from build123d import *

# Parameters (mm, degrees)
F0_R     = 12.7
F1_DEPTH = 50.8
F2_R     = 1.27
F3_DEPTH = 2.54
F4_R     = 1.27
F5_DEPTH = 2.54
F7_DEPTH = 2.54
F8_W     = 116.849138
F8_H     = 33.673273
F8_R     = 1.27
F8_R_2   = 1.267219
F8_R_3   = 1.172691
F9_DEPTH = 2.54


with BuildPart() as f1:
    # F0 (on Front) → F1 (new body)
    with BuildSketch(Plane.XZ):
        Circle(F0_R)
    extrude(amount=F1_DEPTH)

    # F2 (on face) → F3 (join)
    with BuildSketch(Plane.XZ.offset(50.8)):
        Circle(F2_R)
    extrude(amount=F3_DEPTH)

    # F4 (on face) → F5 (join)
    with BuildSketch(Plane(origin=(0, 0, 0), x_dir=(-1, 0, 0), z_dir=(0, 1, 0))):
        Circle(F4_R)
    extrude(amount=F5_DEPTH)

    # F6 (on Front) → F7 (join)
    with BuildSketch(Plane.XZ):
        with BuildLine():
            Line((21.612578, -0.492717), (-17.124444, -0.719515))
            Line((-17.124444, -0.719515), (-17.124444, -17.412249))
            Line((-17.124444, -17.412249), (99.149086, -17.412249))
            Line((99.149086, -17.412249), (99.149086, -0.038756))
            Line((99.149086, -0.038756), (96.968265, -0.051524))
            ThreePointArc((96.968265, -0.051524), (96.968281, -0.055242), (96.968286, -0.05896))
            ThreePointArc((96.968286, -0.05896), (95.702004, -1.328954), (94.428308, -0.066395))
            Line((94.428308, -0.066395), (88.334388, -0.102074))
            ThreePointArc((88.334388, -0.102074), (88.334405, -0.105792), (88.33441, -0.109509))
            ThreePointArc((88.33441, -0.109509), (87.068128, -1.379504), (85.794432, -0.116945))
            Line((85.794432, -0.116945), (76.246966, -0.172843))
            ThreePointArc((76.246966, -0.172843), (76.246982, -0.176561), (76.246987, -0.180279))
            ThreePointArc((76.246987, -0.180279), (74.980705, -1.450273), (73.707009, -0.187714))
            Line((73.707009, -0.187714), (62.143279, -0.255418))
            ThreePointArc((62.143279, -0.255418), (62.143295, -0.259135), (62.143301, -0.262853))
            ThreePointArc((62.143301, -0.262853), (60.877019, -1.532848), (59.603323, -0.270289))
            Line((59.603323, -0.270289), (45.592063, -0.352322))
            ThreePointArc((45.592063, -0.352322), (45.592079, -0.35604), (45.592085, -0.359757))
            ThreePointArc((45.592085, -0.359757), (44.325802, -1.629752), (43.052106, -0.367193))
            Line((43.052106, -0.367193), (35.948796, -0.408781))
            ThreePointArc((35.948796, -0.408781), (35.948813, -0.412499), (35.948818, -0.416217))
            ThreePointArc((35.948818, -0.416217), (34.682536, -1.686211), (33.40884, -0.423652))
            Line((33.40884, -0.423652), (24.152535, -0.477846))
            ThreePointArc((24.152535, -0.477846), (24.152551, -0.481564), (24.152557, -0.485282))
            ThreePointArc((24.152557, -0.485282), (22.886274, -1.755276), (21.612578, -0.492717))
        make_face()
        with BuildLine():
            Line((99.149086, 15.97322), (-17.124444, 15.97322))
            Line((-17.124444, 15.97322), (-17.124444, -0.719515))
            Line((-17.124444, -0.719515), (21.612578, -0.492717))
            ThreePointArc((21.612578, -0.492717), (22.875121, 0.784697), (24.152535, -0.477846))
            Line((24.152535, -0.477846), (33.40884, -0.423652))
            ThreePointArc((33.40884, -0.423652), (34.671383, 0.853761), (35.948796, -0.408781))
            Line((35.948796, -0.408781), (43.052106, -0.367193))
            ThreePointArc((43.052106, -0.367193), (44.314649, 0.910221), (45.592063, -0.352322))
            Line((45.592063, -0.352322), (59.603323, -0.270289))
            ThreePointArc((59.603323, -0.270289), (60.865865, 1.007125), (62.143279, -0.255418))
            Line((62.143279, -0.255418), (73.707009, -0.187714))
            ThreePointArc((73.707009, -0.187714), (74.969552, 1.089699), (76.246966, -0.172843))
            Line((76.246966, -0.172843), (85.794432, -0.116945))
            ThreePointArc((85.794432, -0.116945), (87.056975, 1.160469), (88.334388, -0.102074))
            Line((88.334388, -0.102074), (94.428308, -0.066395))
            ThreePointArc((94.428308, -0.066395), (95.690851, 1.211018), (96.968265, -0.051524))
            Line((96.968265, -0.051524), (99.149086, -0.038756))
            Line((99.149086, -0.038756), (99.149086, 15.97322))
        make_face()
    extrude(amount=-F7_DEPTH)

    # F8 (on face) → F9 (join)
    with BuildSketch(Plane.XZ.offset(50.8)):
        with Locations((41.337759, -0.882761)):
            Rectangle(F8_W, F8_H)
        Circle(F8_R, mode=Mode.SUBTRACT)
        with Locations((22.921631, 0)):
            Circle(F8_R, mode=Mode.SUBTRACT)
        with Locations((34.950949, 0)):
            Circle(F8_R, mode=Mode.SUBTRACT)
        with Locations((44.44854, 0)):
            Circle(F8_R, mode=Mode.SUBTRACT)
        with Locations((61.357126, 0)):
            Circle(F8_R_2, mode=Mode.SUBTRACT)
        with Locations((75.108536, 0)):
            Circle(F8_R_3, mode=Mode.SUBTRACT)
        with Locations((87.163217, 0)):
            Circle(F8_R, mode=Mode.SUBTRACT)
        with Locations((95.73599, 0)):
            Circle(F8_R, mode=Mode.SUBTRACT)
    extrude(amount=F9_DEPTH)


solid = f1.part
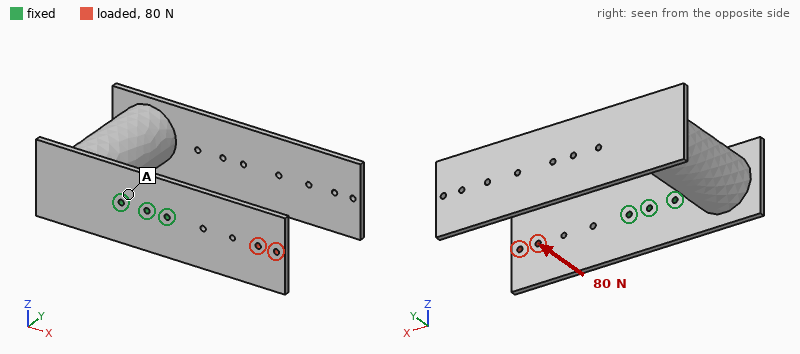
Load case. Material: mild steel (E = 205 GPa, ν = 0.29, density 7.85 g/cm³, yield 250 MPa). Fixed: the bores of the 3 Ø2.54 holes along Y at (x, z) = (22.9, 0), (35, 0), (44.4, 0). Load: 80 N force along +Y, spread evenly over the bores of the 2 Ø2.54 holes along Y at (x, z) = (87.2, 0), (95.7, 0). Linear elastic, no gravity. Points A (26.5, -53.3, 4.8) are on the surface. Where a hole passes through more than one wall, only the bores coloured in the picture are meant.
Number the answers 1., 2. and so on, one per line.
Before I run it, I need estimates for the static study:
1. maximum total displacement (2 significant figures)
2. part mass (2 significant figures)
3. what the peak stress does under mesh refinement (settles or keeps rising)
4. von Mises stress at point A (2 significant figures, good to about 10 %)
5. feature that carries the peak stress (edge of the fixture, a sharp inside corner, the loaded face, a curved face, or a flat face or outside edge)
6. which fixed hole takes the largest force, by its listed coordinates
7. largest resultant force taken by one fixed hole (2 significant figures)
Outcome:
1. 0.41 mm
2. 360 g
3. keeps rising
4. 10 MPa
5. edge of the fixture
6. (44.4, 0)
7. 270 N
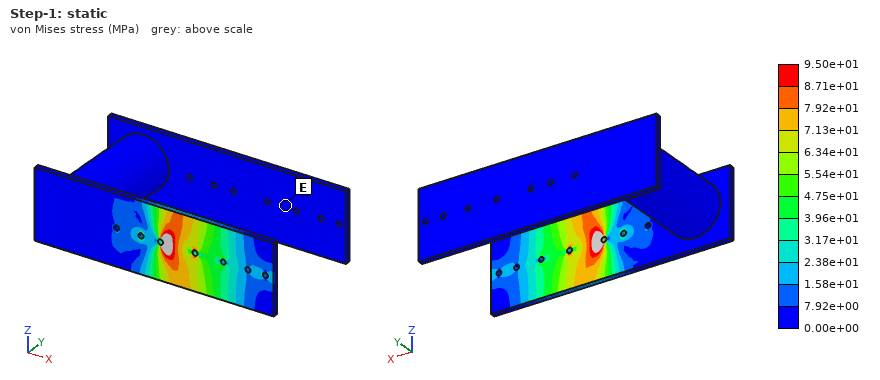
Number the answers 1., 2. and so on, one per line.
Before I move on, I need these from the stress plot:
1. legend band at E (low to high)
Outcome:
1. 0.00e+00 to 7.92e+00 MPa
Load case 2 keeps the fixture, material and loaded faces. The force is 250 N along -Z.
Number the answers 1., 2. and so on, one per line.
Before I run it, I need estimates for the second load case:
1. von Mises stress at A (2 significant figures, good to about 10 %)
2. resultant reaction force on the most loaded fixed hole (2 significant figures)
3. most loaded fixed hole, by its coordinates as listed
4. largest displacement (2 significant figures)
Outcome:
1. 14 MPa
2. 770 N
3. (44.4, 0)
4. 19 µm
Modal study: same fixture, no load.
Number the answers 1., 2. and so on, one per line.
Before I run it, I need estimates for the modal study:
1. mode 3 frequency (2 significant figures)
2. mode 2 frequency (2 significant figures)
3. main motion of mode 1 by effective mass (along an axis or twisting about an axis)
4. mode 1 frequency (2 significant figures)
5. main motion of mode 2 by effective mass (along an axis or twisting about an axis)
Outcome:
1. 310 Hz
2. 260 Hz
3. along X
4. 160 Hz
5. along Z
